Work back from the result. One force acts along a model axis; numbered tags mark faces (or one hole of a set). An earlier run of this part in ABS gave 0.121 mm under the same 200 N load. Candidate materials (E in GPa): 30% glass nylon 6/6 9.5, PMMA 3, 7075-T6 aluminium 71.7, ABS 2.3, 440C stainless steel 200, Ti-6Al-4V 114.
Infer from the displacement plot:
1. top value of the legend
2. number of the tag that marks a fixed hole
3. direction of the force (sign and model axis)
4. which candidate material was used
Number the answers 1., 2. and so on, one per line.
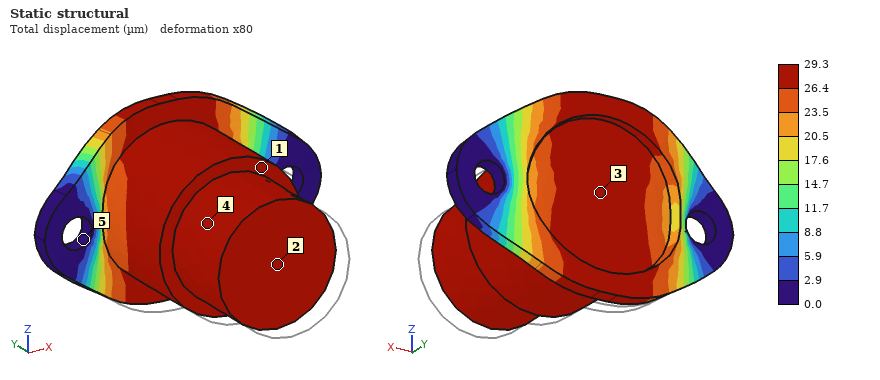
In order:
1. 29.3 µm
2. 5
3. +Y
4. 30% glass nylon 6/6
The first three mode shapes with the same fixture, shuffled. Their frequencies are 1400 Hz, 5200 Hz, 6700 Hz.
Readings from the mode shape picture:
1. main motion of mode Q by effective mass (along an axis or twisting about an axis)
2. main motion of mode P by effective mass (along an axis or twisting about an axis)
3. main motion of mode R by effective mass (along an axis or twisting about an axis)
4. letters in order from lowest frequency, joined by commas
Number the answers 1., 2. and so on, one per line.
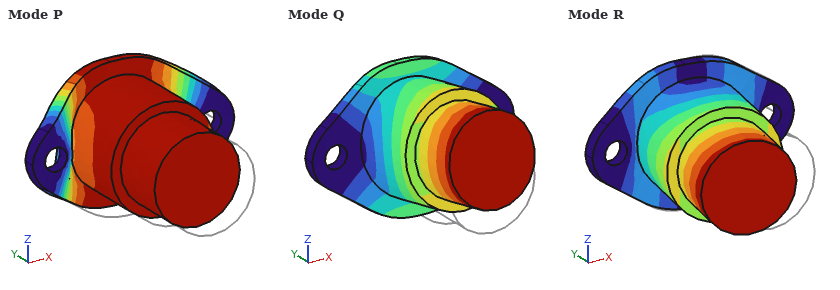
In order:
1. along Z
2. along Y
3. along X
4. Q, R, P
